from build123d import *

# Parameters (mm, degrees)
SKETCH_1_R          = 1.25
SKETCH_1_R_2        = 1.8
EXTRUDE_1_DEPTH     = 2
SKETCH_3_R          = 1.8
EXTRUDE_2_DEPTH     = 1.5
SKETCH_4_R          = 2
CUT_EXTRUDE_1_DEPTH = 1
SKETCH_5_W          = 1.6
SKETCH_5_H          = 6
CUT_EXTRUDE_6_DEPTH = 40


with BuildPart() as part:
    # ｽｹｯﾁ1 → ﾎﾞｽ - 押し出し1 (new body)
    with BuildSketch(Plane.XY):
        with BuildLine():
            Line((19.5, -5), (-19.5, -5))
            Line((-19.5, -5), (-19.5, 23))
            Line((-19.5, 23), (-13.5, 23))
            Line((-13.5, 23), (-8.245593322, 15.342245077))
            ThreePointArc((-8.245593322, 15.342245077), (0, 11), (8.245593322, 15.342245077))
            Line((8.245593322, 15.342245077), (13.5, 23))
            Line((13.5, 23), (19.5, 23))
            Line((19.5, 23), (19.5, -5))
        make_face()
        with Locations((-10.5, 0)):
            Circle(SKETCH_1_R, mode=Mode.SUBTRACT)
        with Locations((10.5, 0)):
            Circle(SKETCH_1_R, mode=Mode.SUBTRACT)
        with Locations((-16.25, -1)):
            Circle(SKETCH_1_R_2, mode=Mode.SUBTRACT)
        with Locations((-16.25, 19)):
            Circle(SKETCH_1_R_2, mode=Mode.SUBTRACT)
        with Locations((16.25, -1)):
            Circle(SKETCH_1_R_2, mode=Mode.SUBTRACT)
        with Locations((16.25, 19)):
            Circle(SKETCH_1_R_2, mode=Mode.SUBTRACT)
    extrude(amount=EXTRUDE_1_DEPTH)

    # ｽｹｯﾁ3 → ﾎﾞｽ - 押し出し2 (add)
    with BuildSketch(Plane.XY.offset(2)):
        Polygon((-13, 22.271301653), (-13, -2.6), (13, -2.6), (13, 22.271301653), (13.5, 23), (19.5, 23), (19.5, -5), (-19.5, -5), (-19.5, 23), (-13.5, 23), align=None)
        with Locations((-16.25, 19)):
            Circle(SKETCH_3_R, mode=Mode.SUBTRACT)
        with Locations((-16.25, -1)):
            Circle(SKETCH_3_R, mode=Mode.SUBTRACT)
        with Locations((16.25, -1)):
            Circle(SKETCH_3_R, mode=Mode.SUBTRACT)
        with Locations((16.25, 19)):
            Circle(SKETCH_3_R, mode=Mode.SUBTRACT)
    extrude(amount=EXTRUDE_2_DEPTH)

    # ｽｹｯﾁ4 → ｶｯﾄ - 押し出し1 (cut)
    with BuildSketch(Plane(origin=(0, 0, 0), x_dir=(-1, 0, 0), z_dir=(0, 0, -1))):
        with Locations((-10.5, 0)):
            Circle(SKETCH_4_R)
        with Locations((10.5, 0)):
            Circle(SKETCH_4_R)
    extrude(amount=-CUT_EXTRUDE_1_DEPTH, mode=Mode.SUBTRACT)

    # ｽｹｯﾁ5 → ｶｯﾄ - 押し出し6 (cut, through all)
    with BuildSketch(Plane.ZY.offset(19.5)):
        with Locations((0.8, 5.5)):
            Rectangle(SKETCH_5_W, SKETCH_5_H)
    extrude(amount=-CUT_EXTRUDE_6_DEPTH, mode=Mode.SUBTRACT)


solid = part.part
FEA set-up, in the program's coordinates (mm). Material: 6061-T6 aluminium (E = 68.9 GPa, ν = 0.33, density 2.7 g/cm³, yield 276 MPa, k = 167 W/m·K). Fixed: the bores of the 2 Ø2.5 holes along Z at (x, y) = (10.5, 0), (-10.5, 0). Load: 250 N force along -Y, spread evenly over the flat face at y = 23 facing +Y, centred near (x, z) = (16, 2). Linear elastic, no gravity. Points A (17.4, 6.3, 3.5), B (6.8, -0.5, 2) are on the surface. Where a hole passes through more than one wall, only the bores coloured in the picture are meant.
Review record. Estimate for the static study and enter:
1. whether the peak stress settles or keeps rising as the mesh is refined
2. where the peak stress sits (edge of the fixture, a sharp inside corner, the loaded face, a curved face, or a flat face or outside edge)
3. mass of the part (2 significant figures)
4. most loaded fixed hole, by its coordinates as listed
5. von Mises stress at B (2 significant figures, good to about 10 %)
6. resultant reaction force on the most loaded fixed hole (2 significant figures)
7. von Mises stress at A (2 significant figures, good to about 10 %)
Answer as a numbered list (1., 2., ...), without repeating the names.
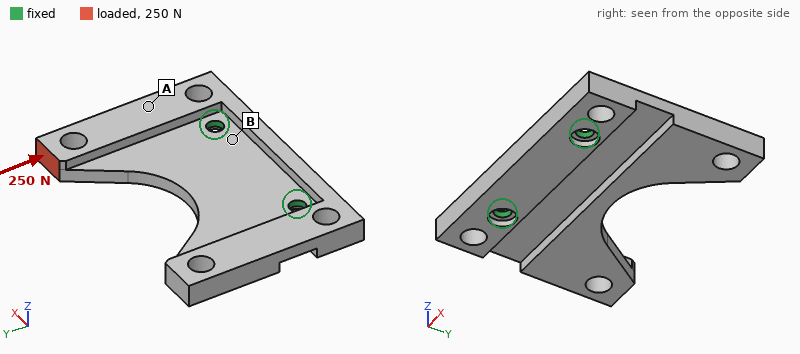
1. keeps rising
2. edge of the fixture
3. 5.0 g
4. (10.5, 0)
5. 7.7 MPa
6. 310 N
7. 17 MPa
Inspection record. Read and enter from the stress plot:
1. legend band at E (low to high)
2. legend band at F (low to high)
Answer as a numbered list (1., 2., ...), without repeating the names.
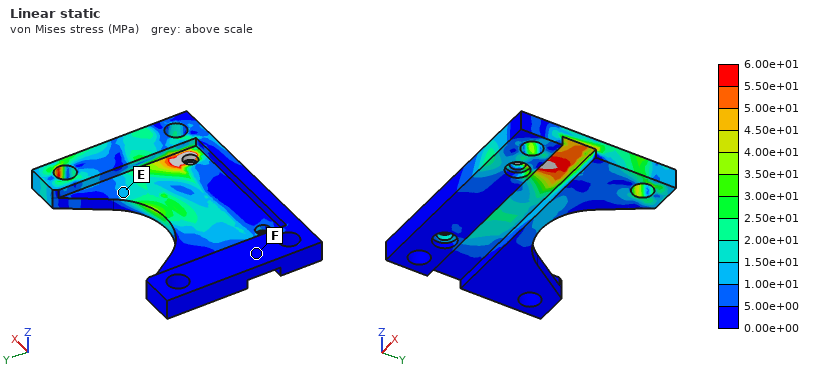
1. 1.00e+01 to 1.50e+01 MPa
2. 0.00e+00 to 5.00e+00 MPa
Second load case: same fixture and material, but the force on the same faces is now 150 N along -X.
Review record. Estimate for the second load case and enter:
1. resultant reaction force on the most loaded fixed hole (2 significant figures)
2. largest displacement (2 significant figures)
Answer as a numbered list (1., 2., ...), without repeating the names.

1. 170 N
2. 86 µm
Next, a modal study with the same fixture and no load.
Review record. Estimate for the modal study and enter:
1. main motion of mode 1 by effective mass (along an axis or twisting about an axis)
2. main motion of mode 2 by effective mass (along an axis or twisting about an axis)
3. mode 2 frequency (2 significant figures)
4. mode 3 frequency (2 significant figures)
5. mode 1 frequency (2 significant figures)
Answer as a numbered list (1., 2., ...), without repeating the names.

1. along Z
2. twisting about Y
3. 2500 Hz
4. 7600 Hz
5. 1900 Hz
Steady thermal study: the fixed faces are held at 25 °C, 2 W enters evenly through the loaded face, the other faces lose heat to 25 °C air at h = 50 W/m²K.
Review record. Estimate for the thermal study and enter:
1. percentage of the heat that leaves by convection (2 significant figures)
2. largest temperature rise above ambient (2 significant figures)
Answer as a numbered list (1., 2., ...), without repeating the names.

1. 16 %
2. 13 K
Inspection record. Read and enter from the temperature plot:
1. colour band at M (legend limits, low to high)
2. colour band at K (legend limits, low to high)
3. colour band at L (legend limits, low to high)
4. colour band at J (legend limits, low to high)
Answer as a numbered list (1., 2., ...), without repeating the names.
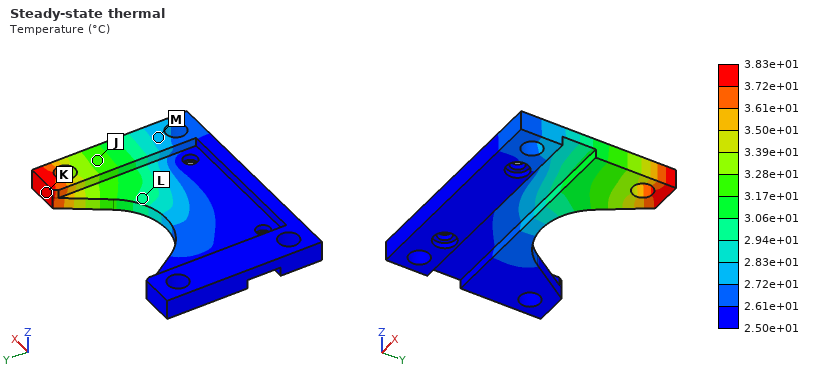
1. 2.72e+01 to 2.83e+01 °C
2. 3.72e+01 to 3.83e+01 °C
3. 2.94e+01 to 3.06e+01 °C
4. 3.17e+01 to 3.28e+01 °C
